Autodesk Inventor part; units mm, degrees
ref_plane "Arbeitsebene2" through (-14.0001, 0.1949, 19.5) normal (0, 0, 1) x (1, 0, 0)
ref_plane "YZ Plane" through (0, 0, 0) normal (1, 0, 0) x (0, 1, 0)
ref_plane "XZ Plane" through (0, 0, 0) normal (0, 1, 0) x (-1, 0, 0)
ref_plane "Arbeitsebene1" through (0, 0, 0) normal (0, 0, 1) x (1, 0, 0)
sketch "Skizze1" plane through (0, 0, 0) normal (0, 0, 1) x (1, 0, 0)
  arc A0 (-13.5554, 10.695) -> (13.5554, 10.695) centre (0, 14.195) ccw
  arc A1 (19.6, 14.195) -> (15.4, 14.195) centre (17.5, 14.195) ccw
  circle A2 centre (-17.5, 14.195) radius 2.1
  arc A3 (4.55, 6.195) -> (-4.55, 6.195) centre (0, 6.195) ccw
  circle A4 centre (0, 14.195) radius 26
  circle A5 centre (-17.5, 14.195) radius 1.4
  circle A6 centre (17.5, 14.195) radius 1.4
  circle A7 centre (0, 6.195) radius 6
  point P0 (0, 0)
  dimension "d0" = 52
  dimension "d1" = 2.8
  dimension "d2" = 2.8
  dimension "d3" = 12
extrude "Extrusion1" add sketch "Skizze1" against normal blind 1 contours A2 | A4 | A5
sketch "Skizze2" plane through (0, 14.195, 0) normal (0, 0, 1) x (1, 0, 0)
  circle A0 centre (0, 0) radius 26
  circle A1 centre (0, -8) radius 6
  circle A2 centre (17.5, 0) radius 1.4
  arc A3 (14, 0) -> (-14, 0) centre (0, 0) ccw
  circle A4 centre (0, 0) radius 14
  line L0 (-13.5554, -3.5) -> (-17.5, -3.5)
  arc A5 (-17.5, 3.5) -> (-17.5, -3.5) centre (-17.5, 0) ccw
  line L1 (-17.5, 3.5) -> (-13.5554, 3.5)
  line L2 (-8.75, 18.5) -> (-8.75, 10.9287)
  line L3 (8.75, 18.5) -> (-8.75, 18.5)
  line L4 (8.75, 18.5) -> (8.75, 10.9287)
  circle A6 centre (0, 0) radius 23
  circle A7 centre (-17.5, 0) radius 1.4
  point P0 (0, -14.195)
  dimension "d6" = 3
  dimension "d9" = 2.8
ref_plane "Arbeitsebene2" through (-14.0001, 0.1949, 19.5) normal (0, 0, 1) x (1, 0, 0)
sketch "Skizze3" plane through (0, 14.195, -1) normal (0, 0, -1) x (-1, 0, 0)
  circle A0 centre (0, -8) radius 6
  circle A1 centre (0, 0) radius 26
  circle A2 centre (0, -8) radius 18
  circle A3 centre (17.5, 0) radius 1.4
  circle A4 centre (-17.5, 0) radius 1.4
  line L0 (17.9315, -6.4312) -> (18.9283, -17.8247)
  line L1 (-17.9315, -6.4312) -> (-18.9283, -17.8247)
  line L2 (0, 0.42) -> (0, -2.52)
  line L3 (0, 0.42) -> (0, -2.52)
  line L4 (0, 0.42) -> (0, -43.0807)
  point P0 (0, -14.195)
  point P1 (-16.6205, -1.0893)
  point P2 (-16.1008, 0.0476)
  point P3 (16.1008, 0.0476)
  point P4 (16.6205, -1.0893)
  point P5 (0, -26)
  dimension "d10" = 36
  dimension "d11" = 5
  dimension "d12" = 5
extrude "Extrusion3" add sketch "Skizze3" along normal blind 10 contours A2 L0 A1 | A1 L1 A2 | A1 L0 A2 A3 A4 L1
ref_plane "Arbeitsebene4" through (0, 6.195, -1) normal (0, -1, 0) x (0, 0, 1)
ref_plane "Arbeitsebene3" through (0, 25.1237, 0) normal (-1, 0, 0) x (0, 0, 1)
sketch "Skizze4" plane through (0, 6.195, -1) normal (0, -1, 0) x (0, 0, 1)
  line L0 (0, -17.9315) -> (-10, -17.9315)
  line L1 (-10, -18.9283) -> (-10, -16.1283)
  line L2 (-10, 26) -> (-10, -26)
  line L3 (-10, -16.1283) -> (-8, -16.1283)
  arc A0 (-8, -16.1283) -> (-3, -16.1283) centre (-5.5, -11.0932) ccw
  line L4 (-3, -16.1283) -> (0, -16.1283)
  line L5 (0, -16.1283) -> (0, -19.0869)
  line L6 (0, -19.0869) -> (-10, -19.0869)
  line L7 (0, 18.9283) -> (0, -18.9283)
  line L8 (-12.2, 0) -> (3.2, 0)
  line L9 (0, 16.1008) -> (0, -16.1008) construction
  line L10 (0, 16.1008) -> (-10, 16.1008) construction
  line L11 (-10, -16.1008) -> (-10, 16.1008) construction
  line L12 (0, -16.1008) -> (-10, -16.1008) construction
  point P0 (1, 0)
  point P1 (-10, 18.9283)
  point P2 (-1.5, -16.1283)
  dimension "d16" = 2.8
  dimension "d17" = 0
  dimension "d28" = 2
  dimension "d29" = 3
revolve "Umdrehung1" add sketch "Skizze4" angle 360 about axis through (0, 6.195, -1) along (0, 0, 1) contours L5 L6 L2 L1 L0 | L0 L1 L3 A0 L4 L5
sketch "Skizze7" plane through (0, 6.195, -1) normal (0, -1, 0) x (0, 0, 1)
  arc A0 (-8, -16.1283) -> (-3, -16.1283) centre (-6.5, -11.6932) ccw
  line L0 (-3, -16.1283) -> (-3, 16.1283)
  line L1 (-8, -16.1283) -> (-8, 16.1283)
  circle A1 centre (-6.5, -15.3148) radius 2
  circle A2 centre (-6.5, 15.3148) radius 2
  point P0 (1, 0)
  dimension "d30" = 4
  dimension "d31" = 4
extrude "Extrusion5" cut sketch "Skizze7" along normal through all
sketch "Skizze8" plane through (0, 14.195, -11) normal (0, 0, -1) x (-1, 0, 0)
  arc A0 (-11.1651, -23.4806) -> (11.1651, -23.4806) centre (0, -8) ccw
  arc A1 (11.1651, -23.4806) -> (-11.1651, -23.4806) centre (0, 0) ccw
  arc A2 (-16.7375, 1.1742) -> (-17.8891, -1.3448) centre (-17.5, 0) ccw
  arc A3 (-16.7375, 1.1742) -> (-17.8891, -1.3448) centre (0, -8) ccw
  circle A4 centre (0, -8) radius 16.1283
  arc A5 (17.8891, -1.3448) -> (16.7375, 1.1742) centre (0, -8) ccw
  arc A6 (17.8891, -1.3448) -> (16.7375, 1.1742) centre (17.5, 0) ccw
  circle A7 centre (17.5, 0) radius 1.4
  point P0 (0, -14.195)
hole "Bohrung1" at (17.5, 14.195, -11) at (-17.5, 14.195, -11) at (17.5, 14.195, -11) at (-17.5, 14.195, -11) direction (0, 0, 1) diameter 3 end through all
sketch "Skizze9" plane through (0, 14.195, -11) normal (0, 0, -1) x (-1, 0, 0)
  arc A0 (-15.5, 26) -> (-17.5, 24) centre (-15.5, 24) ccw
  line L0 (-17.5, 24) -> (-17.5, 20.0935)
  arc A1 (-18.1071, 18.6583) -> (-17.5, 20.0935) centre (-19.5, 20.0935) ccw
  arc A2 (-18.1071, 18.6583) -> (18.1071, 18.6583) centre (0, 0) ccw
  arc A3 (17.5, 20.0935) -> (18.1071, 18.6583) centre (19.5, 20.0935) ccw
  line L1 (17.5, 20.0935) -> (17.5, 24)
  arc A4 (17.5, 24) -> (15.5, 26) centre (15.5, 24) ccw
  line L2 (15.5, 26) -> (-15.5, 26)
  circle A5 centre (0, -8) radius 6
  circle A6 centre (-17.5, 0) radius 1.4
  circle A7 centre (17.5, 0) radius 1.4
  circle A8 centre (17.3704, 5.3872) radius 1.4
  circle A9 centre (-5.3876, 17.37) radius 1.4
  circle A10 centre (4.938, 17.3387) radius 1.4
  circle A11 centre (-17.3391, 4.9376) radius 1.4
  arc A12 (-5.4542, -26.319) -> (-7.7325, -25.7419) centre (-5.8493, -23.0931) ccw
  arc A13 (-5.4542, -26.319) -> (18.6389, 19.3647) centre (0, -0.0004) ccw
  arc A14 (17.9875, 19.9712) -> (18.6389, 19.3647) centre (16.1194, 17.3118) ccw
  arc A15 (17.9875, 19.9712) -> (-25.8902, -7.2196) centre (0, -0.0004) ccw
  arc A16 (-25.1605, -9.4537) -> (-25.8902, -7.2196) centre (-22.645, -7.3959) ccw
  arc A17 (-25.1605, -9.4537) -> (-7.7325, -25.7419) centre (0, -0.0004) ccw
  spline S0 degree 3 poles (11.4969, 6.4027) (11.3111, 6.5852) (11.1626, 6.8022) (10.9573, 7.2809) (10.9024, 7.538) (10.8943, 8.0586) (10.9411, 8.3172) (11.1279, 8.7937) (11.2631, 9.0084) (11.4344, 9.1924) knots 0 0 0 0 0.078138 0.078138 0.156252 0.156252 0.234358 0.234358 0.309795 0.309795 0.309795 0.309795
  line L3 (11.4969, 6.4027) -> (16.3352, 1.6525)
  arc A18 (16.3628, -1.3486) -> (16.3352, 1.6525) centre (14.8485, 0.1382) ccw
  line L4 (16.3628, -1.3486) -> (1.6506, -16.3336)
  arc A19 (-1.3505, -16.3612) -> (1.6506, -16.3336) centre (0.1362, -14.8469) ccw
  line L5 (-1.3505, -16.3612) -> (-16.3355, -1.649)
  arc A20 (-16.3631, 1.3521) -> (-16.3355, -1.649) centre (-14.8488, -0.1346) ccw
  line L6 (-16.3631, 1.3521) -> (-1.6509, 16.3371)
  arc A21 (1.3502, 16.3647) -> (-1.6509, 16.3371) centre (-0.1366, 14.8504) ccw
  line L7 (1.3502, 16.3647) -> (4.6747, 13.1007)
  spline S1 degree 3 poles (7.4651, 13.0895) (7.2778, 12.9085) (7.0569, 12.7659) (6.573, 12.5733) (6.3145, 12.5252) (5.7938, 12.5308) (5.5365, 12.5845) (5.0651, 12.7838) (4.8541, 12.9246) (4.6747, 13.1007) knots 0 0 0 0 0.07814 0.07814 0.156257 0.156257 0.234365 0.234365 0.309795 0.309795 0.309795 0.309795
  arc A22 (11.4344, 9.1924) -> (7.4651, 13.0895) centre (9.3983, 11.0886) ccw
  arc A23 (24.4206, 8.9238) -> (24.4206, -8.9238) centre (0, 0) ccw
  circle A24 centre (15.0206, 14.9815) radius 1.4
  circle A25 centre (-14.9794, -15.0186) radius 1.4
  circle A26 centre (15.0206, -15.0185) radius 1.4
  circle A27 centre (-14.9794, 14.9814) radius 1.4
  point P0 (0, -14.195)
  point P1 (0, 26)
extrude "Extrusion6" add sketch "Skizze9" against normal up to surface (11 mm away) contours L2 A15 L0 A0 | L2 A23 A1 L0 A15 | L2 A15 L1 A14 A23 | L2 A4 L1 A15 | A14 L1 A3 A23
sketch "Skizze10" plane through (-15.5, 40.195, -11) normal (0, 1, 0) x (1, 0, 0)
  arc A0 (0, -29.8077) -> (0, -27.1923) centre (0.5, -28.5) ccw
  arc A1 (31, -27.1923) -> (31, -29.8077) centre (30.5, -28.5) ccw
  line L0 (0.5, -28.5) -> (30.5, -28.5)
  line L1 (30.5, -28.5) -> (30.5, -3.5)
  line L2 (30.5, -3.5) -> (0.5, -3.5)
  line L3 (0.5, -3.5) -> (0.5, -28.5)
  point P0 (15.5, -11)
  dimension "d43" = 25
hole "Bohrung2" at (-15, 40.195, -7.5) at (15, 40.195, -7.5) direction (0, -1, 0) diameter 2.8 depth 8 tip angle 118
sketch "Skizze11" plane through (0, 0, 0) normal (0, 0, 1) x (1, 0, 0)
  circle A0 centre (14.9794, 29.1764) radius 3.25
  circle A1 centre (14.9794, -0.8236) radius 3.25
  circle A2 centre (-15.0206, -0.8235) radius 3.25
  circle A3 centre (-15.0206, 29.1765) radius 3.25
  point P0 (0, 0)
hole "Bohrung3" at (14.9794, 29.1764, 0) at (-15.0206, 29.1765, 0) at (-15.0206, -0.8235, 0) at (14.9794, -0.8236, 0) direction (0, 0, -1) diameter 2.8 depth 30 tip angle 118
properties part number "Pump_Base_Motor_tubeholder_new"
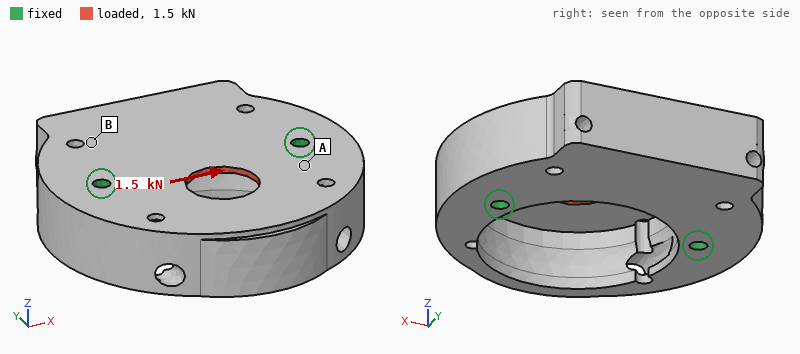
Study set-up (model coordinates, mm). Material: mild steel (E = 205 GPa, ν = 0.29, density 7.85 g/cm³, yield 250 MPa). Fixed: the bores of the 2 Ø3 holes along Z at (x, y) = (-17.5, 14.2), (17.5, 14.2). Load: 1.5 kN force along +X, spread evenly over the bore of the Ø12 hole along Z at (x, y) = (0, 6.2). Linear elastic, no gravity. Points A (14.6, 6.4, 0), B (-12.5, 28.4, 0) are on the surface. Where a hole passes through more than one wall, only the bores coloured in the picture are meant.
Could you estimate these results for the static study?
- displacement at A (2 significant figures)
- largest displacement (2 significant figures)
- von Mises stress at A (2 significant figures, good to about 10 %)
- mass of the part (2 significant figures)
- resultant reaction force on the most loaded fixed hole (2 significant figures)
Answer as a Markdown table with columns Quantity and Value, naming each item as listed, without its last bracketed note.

| Quantity | Value |
|---|---|
| displacement at A | 2.2 µm |
| largest displacement | 5.7 µm |
| von Mises stress at A | 37 MPa |
| mass of the part | 120 g |
| resultant reaction force on the most loaded fixed hole | 800 N |
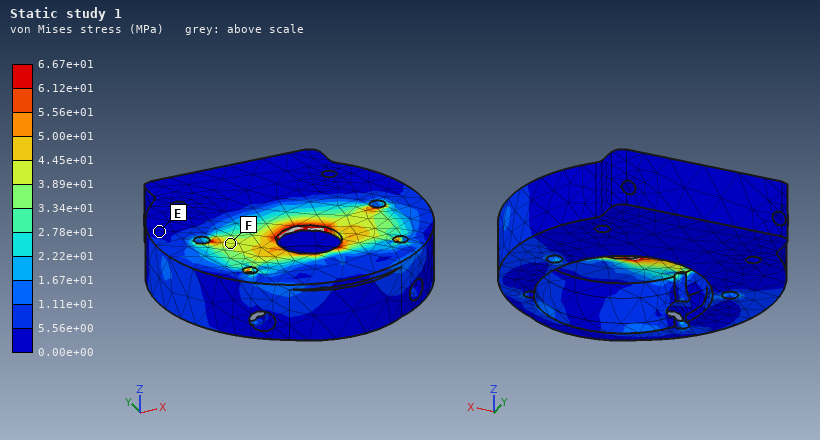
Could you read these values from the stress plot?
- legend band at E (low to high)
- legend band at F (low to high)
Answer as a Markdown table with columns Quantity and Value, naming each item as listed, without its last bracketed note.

| Quantity | Value |
|---|---|
| legend band at E | 0.00e+00 to 5.56e+00 MPa |
| legend band at F | 3.89e+01 to 4.45e+01 MPa |
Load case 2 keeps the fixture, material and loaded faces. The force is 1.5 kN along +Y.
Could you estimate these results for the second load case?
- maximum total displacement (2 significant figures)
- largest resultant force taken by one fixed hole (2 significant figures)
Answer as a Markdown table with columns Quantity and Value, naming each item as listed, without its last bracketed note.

| Quantity | Value |
|---|---|
| maximum total displacement | 4.9 µm |
| largest resultant force taken by one fixed hole | 750 N |
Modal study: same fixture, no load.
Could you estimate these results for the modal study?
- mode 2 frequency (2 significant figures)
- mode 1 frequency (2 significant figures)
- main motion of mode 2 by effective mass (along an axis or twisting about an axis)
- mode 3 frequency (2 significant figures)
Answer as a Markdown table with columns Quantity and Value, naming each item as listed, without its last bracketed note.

| Quantity | Value |
|---|---|
| mode 2 frequency | 9900 Hz |
| mode 1 frequency | 8800 Hz |
| main motion of mode 2 by effective mass | along Z |
| mode 3 frequency | 12 kHz |
